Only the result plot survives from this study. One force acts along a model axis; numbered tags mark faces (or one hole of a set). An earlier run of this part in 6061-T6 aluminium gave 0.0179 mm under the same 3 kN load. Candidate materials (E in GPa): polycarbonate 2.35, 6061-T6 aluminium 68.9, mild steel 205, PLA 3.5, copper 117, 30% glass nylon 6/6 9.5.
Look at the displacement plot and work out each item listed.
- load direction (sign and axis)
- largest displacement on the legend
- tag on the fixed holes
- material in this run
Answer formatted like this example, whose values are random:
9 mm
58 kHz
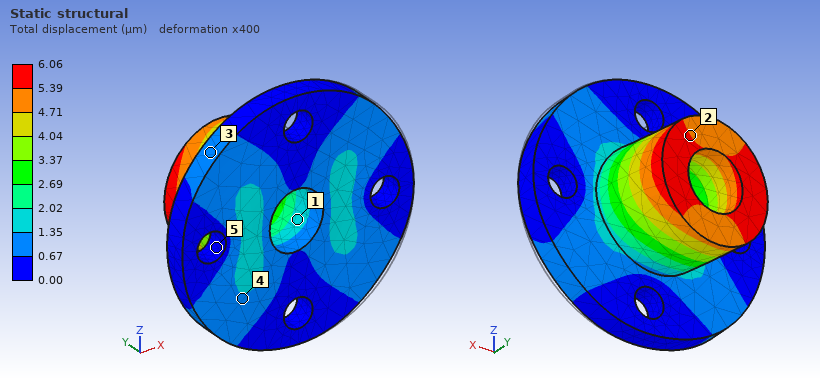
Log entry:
-X
6.06 µm
5
mild steel
